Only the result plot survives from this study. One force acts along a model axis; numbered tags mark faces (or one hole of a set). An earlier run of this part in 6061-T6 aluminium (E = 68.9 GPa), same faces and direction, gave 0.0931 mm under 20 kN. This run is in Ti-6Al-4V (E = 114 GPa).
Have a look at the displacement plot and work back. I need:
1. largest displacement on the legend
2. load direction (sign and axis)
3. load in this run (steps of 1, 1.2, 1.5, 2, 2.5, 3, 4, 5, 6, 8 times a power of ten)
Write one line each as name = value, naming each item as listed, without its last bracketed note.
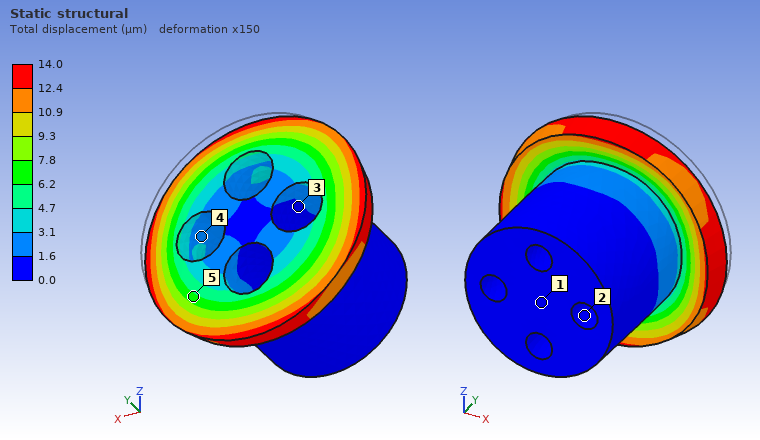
largest displacement on the legend = 14.0 µm
load direction = -Y
load in this run = 5 kN
